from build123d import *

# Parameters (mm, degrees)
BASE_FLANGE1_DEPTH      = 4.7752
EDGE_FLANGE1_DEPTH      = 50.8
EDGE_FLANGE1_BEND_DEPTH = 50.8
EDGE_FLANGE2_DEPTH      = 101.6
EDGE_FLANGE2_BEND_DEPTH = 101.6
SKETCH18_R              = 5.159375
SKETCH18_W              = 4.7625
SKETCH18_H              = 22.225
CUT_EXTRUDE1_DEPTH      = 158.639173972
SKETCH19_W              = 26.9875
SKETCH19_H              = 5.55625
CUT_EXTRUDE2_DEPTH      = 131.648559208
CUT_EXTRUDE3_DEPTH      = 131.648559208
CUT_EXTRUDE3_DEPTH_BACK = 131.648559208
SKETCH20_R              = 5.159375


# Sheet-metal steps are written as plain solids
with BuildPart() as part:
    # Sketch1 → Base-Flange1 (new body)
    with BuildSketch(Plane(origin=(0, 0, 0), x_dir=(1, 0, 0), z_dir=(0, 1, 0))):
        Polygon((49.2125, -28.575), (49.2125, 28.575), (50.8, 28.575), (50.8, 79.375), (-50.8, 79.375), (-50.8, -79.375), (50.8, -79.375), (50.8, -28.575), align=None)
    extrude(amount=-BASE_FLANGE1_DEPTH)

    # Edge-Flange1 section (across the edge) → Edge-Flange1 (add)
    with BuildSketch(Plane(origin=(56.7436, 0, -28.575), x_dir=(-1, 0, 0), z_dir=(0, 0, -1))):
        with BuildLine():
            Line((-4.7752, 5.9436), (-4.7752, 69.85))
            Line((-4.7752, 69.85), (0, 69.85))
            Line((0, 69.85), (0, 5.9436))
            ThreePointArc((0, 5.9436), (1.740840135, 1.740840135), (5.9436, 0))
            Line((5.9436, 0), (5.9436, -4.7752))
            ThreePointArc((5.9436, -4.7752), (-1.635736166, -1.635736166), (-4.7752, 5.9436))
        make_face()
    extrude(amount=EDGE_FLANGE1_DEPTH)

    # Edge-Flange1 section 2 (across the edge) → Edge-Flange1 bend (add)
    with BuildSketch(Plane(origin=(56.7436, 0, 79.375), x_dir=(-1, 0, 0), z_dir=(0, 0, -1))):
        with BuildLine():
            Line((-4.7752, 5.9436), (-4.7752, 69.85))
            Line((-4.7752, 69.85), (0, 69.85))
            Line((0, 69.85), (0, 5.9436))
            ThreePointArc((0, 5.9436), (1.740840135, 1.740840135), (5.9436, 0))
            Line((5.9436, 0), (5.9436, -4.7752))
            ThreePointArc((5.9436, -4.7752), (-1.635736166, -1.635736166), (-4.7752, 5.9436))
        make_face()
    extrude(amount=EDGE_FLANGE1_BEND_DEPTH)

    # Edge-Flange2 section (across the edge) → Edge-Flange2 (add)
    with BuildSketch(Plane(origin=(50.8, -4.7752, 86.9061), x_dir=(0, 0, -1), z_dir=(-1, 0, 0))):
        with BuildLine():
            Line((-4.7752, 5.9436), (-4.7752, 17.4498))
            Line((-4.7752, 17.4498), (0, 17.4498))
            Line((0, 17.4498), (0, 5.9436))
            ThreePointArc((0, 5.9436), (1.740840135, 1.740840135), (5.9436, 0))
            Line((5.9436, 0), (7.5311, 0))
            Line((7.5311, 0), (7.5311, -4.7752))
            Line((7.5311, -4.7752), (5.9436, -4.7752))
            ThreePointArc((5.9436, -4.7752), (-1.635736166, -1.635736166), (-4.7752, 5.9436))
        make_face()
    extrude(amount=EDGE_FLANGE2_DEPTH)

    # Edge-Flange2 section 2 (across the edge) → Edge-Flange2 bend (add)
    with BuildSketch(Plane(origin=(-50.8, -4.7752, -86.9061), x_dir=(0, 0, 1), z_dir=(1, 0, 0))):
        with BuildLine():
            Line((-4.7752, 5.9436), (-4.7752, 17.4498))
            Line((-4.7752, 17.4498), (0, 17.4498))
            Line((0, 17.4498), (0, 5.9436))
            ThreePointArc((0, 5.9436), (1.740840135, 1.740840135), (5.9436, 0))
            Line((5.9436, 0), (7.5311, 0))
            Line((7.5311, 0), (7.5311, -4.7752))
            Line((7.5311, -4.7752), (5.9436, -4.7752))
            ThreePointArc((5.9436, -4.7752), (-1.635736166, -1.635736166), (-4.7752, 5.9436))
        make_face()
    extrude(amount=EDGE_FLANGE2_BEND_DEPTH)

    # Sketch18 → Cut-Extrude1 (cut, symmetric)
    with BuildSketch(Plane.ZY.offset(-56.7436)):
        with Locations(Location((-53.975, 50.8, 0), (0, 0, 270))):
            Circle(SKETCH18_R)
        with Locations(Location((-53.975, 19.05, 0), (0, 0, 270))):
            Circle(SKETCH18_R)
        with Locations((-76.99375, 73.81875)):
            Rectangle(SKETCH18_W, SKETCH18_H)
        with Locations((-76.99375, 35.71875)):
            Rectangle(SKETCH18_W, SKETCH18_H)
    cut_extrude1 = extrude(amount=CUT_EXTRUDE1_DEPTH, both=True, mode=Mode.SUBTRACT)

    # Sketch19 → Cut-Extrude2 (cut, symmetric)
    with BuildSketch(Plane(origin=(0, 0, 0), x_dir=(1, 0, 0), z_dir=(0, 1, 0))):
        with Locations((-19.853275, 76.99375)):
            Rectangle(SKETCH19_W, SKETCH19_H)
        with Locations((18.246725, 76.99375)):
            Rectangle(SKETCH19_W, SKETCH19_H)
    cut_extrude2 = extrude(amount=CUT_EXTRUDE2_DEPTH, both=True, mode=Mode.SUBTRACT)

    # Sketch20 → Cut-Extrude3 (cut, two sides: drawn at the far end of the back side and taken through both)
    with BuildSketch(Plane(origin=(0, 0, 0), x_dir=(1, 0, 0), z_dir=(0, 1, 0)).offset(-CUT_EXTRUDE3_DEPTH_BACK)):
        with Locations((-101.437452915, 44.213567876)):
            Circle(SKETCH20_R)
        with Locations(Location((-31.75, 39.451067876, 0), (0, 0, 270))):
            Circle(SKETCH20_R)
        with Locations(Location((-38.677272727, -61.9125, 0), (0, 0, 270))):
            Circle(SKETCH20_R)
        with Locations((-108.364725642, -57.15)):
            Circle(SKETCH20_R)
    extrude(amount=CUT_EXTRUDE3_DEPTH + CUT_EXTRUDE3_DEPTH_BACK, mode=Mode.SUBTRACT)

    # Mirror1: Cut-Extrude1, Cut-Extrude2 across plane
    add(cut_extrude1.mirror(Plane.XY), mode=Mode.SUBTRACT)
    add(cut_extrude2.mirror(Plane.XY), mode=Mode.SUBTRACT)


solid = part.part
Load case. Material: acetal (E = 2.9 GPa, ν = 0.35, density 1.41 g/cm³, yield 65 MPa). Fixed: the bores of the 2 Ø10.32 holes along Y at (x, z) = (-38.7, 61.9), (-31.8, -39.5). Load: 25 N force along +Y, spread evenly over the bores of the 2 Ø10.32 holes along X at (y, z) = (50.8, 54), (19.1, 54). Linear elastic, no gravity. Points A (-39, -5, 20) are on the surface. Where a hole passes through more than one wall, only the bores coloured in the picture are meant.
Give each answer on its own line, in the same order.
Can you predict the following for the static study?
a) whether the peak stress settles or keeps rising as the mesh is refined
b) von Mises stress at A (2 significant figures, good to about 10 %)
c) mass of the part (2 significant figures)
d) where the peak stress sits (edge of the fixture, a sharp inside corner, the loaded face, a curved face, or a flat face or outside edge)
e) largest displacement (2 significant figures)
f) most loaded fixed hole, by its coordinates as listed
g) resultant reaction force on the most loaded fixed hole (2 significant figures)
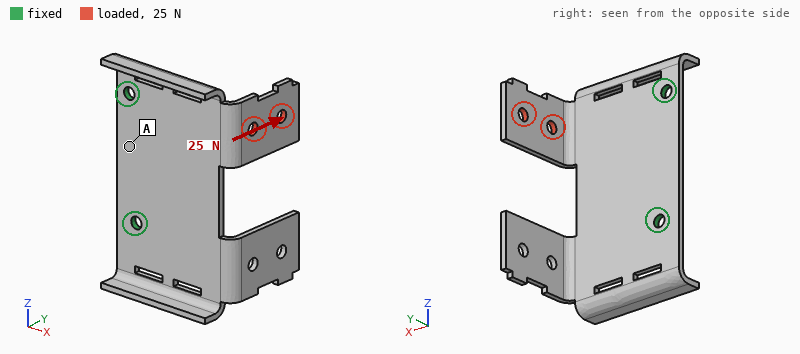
keeps rising
0.69 MPa
190 g
edge of the fixture
2.4 mm
(-38.7, 61.9)
22 N
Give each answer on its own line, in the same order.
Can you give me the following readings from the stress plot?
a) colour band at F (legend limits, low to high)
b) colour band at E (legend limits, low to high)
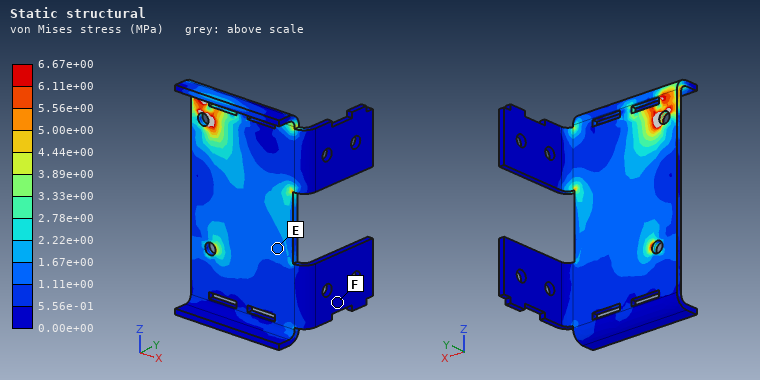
0.00e+00 to 5.56e-01 MPa
1.11e+00 to 1.67e+00 MPa
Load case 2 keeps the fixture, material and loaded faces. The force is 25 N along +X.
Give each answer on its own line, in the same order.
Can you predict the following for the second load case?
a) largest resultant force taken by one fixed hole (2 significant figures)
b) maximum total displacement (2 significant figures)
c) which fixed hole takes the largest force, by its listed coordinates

25 N
2.7 mm
(-38.7, 61.9)
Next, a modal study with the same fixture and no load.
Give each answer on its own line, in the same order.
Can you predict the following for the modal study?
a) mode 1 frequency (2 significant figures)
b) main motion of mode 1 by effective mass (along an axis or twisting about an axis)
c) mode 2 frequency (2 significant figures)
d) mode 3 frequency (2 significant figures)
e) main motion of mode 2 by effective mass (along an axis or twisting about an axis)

79 Hz
along Y
96 Hz
140 Hz
twisting about X
